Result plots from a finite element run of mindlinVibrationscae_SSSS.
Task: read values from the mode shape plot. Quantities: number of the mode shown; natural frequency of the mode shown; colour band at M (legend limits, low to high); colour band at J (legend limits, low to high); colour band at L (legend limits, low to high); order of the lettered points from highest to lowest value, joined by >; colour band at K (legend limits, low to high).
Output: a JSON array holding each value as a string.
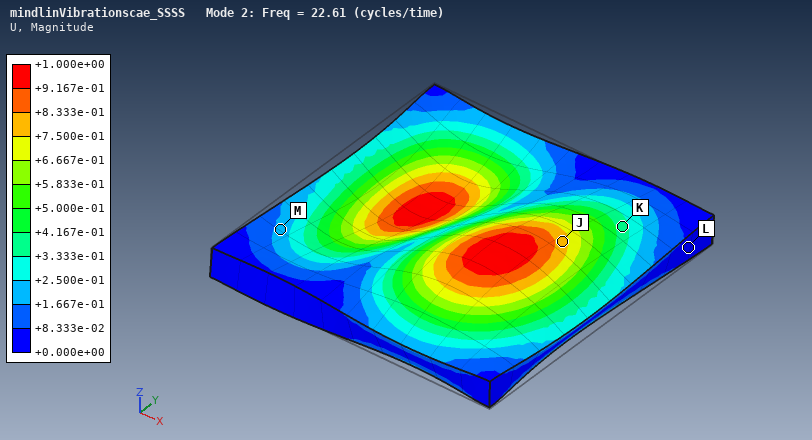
["2", "22.61", "+1.667e-01 to +2.500e-01", "+7.500e-01 to +8.333e-01", "+0.000e+00 to +8.333e-02", "J > K > M > L", "+3.333e-01 to +4.167e-01"]
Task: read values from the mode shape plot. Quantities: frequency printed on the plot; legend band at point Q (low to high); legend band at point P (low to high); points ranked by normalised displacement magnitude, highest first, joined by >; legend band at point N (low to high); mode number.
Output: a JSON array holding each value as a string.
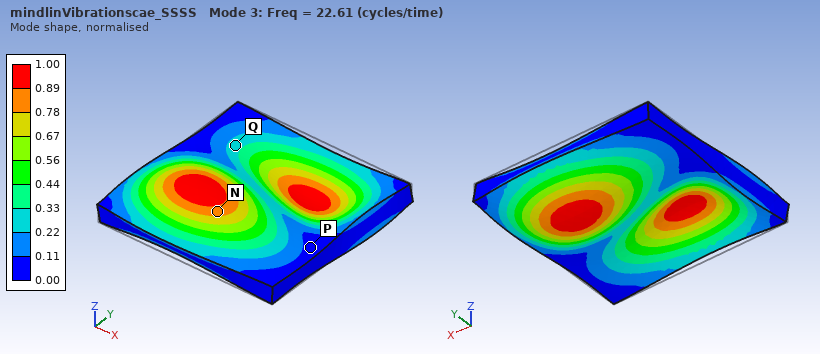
["22.61", "0.22 to 0.33", "0.00 to 0.11", "N > Q > P", "0.78 to 0.89", "3"]
